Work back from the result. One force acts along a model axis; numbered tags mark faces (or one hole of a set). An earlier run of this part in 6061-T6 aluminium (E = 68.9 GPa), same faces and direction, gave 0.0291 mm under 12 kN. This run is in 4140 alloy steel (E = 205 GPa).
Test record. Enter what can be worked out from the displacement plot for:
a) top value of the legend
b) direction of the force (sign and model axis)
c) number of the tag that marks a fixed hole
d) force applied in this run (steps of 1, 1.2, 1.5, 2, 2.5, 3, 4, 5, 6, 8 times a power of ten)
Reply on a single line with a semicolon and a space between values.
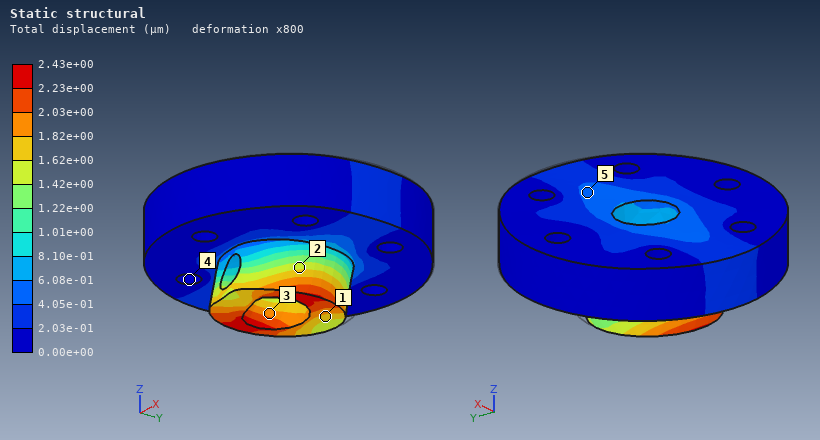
2.43e+00 µm; -X; 4; 3 kN
